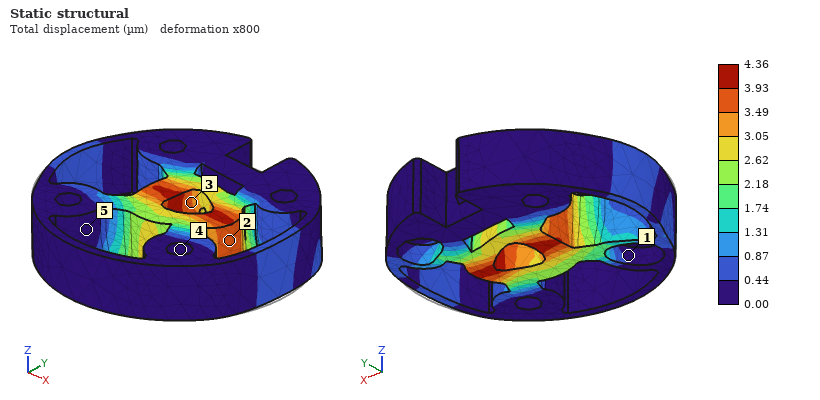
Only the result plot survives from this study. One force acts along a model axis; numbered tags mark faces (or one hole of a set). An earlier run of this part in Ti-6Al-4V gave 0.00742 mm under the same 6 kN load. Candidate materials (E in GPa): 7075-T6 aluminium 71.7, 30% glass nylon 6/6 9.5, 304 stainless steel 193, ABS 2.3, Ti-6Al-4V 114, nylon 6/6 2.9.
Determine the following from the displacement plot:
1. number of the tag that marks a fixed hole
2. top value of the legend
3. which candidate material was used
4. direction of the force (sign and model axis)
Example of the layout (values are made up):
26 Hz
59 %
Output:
4
4.36 µm
304 stainless steel
+X
